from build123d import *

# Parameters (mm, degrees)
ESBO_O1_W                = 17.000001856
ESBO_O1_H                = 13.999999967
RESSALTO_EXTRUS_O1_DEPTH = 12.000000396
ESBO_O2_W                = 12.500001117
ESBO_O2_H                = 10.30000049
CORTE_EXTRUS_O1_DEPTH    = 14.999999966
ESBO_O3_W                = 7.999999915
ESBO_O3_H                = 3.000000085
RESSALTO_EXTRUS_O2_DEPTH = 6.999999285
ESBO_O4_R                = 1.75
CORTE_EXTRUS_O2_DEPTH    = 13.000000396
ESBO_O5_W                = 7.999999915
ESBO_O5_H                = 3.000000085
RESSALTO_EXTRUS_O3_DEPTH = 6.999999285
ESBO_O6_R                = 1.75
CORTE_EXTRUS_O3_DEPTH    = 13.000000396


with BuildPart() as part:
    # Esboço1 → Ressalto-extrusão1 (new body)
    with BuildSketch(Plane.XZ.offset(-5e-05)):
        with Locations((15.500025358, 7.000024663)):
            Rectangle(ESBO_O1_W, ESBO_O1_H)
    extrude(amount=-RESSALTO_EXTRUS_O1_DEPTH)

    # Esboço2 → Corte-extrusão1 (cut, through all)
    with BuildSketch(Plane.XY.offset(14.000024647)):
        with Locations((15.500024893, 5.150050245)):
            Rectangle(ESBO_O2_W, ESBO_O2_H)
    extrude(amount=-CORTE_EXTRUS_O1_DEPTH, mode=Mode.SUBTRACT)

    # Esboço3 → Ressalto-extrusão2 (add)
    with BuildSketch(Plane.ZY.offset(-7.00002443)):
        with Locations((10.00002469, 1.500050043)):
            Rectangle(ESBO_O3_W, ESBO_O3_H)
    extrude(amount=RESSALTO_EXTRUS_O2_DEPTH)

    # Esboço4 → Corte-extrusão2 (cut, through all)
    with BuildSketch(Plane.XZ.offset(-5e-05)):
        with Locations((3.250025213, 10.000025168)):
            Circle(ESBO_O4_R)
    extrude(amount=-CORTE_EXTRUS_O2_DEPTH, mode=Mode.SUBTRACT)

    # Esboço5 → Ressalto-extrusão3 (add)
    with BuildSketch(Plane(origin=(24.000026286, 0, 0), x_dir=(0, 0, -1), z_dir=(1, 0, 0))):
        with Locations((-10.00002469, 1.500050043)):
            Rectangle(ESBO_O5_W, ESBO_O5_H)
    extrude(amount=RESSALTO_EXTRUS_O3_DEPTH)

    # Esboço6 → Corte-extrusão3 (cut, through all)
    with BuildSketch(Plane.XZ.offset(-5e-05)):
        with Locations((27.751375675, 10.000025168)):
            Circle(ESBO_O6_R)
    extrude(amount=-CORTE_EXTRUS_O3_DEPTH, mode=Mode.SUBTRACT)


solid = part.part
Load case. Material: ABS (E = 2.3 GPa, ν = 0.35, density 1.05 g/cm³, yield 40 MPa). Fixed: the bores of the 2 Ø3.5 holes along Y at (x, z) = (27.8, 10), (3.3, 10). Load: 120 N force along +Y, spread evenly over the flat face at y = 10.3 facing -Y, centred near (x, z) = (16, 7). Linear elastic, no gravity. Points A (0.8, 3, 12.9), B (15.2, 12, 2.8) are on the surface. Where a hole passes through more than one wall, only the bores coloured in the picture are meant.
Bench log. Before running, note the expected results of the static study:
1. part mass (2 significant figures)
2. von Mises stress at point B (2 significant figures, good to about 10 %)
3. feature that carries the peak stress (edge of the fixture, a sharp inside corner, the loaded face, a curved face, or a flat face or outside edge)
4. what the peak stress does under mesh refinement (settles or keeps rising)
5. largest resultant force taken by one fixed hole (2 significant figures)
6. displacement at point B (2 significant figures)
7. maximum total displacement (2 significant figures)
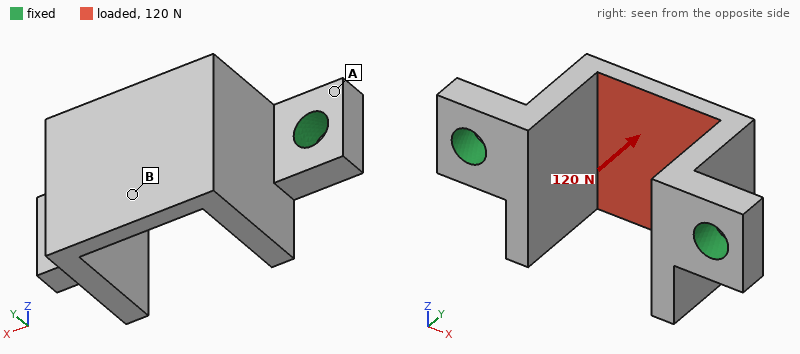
1.4 g
14 MPa
edge of the fixture
keeps rising
66 N
0.25 mm
0.30 mm
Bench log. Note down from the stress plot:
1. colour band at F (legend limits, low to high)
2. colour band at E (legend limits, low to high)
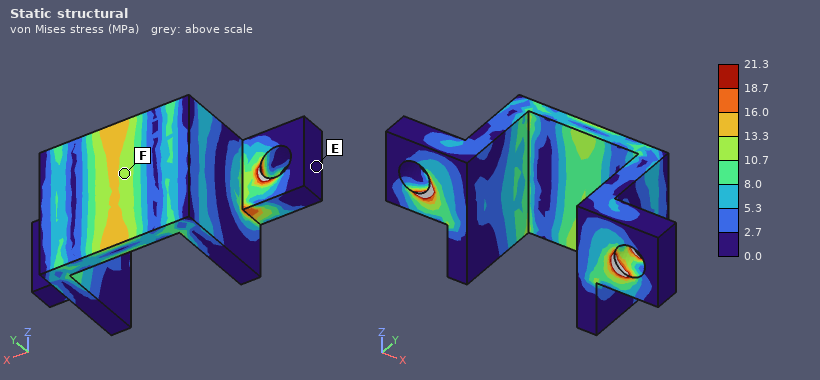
10.7 to 13.3 MPa
0.0 to 2.7 MPa
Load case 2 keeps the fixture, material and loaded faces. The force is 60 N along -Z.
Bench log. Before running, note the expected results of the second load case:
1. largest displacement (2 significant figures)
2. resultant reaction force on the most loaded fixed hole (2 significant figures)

0.26 mm
30 N
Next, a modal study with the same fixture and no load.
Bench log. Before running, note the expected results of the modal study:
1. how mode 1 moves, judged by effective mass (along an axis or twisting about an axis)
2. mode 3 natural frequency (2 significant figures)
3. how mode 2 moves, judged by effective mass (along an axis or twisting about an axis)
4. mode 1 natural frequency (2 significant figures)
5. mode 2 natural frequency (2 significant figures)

along Z
4500 Hz
along X
3000 Hz
3500 Hz
